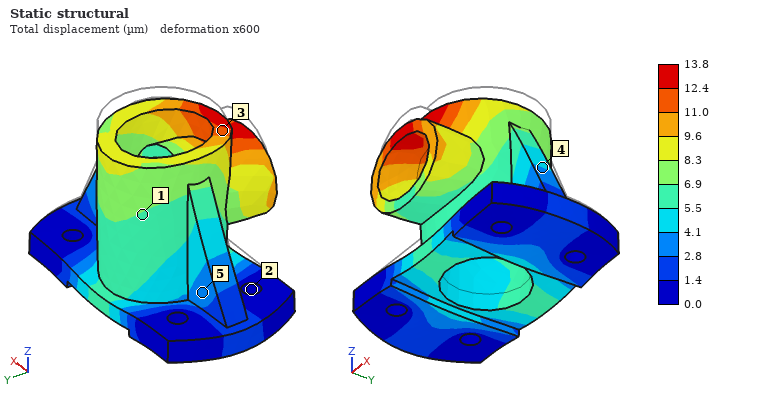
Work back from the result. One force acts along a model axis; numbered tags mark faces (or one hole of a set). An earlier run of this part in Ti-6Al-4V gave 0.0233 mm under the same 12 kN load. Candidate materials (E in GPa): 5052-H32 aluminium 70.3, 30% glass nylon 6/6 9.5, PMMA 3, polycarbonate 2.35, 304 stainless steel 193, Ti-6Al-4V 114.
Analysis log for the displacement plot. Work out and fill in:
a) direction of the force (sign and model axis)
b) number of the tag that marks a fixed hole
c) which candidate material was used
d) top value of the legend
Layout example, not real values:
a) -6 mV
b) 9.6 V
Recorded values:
a) -Z
b) 2
c) 304 stainless steel
d) 13.8 µm
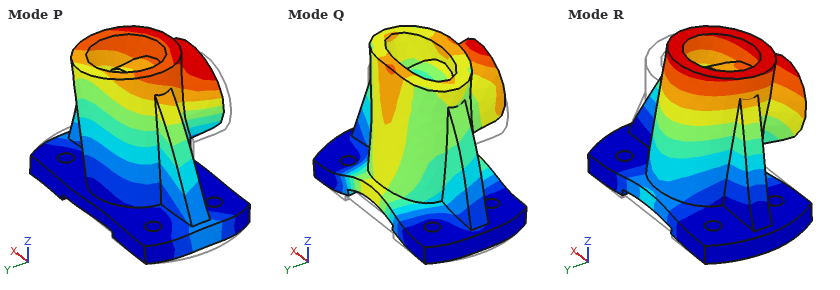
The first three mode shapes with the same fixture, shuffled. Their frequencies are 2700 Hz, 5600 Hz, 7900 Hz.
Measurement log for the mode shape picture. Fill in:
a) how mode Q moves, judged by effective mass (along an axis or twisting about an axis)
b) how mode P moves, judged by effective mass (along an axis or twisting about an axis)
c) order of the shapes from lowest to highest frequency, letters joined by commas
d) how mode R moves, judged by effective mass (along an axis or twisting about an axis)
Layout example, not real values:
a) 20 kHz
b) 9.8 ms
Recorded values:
a) along Z
b) along X
c) R, P, Q
d) along Y
